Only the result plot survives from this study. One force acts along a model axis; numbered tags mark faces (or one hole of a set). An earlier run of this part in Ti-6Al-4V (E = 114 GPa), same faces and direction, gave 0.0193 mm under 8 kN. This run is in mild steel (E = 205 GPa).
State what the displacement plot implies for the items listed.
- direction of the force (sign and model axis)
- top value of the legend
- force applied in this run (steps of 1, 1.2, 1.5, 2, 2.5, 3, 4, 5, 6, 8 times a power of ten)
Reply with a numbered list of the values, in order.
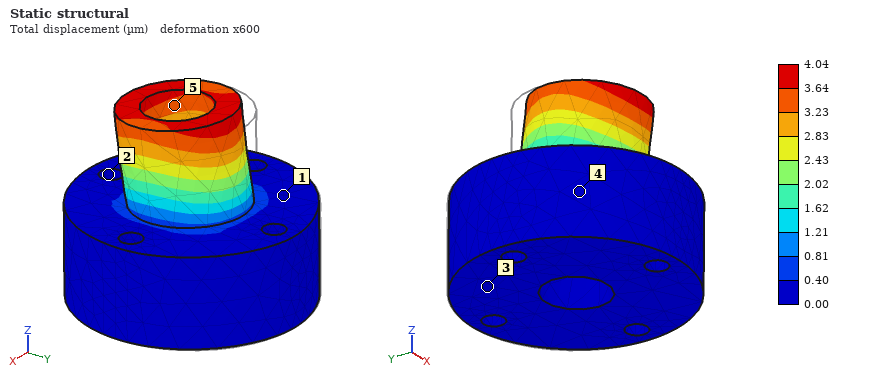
1. -Y
2. 4.04 µm
3. 3 kN
